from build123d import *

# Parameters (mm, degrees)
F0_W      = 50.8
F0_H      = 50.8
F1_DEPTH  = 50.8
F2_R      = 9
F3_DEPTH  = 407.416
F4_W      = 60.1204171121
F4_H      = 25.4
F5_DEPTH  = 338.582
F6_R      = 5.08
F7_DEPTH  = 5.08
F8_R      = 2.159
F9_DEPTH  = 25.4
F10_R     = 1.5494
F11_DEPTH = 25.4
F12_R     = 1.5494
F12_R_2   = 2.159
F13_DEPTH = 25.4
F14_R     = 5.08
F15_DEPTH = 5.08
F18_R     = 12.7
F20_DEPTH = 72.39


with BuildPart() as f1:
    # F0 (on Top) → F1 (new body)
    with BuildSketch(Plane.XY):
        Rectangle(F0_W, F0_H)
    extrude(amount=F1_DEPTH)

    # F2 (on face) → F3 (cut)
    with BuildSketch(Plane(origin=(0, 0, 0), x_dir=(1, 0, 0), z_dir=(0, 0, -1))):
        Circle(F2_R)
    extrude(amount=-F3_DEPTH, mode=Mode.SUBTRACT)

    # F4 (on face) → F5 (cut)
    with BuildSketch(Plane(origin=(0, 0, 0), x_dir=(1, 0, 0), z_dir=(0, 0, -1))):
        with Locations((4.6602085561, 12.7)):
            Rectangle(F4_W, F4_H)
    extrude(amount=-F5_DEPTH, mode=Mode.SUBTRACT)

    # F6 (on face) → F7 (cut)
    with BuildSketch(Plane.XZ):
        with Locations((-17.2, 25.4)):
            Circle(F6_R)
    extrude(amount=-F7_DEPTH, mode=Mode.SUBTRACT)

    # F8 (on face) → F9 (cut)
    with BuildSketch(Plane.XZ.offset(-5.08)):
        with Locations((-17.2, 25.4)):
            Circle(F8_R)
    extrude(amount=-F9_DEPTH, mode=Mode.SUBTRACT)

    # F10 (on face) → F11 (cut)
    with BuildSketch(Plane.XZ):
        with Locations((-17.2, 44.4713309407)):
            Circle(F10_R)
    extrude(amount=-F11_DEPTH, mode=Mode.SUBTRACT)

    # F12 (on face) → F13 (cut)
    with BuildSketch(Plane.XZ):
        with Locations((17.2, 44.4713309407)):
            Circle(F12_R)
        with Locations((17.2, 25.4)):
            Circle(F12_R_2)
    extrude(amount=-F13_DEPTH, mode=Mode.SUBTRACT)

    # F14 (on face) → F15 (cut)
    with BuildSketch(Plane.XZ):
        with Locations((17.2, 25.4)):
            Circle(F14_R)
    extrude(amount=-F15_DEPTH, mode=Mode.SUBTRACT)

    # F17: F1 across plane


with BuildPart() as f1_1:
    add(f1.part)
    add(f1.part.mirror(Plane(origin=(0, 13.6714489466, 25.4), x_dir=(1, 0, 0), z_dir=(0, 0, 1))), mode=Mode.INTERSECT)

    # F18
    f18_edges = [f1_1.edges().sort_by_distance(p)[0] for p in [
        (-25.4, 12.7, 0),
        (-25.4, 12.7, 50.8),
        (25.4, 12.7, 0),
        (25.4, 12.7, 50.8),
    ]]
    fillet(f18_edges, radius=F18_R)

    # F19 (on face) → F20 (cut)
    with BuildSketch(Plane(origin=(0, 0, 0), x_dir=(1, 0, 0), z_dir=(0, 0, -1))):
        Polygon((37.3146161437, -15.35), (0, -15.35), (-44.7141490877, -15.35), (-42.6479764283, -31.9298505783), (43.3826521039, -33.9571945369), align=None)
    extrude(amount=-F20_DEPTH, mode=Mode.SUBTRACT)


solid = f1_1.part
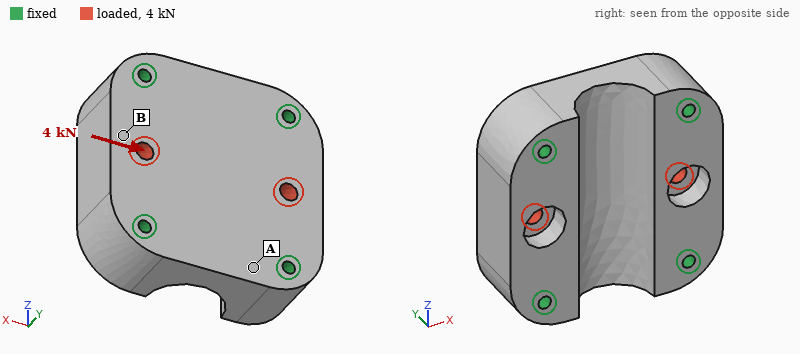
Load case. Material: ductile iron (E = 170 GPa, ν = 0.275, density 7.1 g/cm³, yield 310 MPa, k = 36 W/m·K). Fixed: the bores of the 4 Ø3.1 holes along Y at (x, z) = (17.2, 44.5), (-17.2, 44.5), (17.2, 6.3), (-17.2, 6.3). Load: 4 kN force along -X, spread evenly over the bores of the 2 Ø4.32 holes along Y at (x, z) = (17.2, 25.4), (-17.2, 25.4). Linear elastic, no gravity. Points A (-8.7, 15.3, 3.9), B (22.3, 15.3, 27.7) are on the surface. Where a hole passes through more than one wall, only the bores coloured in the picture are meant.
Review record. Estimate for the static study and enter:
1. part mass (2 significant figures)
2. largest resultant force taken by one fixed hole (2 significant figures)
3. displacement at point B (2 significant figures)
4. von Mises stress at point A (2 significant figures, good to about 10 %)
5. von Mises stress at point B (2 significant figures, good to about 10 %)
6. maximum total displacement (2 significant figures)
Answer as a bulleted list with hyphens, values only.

- 210 g
- 1.0 kN
- 1.7 µm
- 3.5 MPa
- 11 MPa
- 2.0 µm
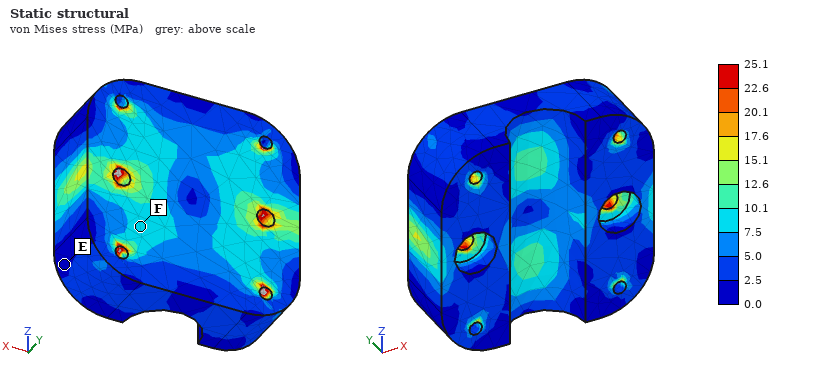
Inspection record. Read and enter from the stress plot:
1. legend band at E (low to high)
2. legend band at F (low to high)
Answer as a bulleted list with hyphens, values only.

- 0.0 to 2.5 MPa
- 7.5 to 10.1 MPa
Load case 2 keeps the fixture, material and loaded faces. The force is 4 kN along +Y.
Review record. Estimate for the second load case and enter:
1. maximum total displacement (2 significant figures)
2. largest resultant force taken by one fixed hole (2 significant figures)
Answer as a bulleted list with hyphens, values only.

- 3.0 µm
- 1.0 kN
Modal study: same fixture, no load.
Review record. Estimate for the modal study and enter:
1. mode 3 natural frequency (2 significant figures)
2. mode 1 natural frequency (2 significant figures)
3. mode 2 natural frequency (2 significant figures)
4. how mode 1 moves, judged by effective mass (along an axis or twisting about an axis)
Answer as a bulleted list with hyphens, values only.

- 31 kHz
- 23 kHz
- 28 kHz
- along Y
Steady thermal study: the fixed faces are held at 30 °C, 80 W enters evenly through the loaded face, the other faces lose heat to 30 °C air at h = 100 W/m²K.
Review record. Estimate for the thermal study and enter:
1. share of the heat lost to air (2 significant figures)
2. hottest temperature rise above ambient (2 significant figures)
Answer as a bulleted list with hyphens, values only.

- 15 %
- 51 K
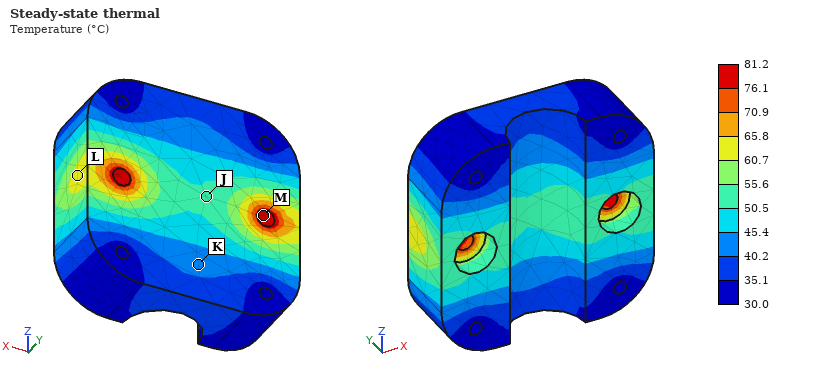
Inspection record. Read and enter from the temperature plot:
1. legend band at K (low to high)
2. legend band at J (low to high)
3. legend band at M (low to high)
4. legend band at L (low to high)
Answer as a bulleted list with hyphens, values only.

- 40.2 to 45.4 °C
- 50.5 to 55.6 °C
- 76.1 to 81.2 °C
- 60.7 to 65.8 °C
